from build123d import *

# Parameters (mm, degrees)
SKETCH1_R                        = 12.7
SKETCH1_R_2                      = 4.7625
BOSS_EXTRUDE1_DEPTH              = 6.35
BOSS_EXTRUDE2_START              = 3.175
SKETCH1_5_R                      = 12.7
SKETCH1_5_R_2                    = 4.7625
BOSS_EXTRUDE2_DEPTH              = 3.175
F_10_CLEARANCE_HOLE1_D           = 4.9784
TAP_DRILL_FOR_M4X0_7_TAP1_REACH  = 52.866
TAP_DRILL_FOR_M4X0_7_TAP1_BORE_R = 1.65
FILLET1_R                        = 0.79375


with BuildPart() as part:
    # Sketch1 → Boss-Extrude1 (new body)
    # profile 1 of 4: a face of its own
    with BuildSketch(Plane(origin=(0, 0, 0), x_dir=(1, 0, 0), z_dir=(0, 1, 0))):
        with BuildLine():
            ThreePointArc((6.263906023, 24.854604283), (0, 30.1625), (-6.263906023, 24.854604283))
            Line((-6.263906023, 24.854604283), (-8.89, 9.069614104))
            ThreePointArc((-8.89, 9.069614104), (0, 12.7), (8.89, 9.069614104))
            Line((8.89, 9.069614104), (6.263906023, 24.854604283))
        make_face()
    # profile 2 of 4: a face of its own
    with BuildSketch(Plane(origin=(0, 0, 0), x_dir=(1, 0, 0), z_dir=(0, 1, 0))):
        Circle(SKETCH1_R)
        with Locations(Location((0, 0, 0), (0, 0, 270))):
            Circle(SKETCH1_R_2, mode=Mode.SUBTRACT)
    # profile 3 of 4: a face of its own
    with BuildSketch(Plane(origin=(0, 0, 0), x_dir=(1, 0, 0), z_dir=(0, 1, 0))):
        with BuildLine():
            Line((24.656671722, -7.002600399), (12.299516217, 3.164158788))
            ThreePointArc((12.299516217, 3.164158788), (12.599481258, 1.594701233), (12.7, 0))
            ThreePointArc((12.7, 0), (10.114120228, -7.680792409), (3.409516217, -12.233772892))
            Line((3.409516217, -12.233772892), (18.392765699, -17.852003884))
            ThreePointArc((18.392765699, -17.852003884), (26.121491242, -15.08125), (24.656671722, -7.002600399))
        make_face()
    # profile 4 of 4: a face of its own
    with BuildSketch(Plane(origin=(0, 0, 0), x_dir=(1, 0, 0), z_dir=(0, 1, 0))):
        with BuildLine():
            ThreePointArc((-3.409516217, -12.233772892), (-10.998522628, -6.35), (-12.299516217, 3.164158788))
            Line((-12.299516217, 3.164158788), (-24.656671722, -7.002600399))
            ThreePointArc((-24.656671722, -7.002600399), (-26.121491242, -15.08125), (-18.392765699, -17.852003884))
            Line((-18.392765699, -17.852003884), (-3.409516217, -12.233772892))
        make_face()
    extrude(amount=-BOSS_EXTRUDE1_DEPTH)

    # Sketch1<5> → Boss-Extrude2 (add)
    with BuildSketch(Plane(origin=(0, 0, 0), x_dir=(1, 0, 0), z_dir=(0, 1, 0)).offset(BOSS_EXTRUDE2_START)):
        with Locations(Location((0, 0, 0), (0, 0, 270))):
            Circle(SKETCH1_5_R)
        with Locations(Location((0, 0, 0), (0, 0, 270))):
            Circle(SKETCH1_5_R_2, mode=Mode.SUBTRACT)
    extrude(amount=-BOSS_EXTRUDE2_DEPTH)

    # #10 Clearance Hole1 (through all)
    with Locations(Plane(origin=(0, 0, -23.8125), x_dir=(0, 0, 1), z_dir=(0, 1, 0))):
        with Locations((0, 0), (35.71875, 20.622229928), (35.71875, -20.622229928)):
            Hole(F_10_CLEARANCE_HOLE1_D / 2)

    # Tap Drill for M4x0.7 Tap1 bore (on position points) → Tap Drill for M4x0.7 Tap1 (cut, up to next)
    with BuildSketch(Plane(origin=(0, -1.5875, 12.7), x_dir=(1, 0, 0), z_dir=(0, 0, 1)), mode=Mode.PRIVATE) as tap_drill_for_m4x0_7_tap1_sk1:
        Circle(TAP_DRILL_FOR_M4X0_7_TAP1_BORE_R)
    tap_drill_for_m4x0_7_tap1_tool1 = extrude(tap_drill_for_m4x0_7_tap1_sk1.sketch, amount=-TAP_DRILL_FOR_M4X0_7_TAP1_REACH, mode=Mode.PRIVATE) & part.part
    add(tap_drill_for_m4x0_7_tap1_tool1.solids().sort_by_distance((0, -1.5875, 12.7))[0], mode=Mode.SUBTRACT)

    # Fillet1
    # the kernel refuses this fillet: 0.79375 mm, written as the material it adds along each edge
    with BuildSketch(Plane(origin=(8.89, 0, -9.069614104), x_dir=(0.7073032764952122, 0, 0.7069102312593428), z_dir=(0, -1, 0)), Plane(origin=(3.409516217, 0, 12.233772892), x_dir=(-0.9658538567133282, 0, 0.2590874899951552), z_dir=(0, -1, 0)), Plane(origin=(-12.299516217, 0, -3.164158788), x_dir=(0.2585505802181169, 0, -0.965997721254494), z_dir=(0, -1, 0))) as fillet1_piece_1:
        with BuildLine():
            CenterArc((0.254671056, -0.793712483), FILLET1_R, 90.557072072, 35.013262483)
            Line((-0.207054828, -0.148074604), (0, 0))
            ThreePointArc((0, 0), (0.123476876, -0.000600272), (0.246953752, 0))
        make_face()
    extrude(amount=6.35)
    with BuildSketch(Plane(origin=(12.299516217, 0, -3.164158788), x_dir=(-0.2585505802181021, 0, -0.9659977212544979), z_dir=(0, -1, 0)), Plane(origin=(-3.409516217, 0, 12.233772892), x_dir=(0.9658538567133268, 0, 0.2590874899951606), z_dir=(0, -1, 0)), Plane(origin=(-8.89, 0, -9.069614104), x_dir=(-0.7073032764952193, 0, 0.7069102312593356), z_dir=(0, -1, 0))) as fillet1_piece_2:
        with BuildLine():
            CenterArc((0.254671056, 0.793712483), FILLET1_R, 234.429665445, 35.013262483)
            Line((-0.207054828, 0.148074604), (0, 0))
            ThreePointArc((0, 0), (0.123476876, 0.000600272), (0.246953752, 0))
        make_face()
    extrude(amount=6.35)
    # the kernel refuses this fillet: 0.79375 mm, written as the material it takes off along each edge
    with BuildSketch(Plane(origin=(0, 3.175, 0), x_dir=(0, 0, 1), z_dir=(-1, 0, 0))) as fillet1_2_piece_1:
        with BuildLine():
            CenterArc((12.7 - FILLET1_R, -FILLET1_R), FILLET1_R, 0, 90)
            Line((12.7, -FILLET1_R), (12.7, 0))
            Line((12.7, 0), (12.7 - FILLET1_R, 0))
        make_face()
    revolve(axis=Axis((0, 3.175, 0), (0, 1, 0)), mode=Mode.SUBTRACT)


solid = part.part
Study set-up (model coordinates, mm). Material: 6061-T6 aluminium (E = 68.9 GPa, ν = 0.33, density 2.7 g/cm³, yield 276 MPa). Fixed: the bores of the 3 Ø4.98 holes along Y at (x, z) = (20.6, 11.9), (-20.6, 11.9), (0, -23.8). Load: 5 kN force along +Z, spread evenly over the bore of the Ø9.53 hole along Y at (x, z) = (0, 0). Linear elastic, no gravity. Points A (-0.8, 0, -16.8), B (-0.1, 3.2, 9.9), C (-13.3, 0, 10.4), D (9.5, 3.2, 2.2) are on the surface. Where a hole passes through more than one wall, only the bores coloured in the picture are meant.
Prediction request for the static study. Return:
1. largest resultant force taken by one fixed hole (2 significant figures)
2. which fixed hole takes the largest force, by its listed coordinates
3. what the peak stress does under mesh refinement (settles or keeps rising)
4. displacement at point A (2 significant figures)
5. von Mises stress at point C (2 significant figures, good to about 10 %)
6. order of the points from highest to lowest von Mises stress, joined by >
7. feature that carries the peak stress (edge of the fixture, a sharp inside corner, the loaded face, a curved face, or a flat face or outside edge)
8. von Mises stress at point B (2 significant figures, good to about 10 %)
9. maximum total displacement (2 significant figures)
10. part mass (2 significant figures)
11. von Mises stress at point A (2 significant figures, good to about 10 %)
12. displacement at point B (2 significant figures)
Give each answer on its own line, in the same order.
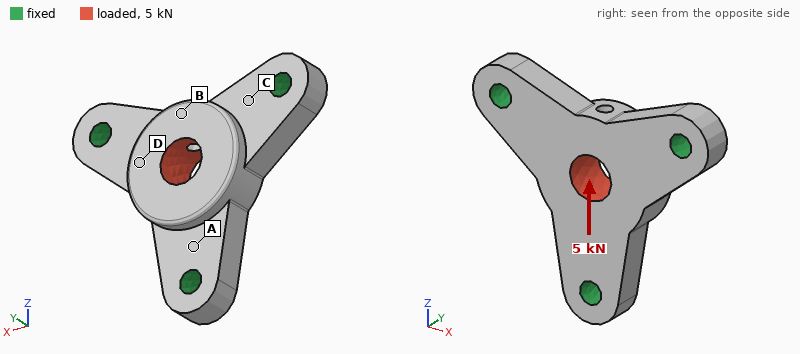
2.7 kN
(0, -23.8)
keeps rising
2.6 µm
23 MPa
A > C > B > D
a sharp inside corner
13 MPa
15 µm
23 g
40 MPa
14 µm
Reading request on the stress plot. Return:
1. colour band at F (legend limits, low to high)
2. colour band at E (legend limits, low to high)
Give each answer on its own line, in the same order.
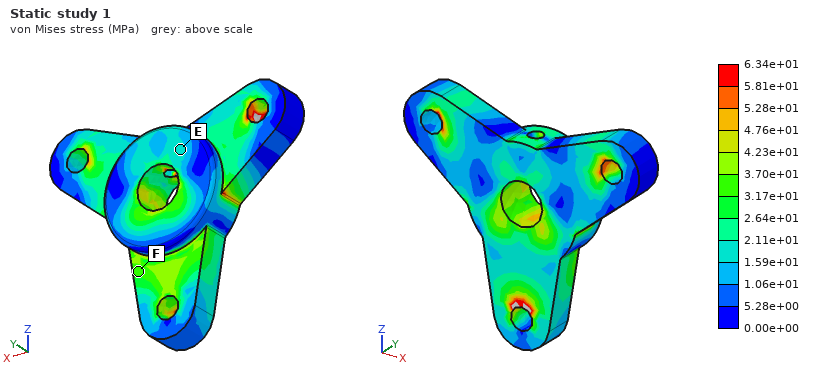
3.17e+01 to 3.70e+01 MPa
1.59e+01 to 2.11e+01 MPa
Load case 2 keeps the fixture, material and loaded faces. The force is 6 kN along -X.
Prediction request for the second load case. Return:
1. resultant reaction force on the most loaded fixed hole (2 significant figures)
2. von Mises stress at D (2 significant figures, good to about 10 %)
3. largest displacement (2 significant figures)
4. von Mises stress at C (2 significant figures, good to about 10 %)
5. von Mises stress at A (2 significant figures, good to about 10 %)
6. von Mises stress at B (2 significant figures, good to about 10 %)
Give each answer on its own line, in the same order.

2.9 kN
22 MPa
18 µm
41 MPa
24 MPa
27 MPa
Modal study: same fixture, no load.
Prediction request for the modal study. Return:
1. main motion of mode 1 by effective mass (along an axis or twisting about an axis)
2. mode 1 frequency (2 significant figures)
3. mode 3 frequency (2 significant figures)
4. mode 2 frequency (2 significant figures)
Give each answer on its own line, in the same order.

along Y
17 kHz
27 kHz
27 kHz
